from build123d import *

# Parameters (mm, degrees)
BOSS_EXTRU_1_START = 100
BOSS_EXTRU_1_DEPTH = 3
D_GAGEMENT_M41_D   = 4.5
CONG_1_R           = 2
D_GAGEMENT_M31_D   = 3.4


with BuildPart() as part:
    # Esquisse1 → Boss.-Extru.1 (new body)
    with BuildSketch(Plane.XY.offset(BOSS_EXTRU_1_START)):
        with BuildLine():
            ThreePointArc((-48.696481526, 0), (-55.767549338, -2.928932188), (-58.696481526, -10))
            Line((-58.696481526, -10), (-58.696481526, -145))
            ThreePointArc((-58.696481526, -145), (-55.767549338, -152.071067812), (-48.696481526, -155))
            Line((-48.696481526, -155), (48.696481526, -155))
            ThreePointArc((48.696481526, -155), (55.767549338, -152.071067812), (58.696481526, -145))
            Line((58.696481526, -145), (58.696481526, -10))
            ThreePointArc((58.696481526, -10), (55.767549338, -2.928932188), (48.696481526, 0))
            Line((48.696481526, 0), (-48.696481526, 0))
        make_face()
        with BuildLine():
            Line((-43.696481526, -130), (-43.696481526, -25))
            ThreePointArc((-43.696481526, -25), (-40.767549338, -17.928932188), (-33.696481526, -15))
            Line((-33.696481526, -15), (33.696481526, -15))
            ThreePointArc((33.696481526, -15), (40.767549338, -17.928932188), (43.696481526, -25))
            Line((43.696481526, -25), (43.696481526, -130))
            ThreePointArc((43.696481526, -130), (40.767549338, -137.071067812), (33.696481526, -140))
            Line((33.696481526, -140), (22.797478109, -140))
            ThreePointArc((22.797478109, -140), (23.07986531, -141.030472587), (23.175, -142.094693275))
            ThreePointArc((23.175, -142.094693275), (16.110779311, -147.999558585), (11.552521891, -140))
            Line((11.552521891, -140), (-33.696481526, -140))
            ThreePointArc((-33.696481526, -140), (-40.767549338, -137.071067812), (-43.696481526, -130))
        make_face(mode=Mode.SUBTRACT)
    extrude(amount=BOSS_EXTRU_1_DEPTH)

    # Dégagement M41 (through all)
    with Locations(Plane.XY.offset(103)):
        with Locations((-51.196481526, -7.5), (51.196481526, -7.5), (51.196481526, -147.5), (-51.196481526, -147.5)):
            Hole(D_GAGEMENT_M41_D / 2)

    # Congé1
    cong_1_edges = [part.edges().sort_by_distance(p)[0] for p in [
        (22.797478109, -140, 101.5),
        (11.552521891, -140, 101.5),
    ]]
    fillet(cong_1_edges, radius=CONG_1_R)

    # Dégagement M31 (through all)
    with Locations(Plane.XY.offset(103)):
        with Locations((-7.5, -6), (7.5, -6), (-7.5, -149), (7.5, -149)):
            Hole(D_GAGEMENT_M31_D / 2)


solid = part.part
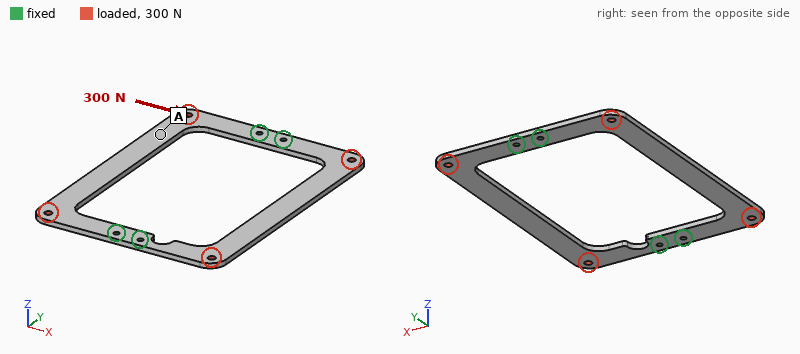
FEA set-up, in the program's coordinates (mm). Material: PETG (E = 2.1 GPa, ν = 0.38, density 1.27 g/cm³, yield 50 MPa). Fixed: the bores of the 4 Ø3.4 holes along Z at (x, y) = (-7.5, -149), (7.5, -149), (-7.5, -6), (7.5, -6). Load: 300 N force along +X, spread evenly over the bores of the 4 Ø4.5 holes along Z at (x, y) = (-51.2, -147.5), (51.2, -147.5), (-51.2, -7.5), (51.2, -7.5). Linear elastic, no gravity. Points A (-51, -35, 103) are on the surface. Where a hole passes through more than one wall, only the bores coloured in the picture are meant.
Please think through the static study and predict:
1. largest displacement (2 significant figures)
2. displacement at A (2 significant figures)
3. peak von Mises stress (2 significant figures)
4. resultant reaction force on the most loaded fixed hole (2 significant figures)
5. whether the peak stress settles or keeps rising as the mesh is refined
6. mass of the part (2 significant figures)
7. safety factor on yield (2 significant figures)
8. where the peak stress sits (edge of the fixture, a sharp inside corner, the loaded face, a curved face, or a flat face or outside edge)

72 µm
21 µm
9.2 MPa
78 N
settles
27 g
5.5
a curved face
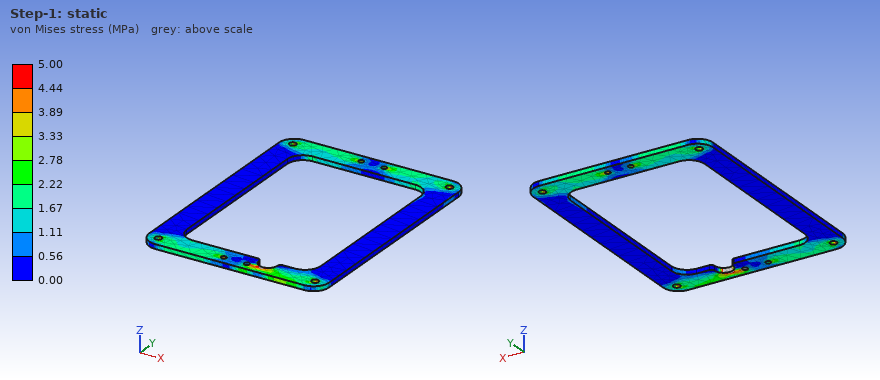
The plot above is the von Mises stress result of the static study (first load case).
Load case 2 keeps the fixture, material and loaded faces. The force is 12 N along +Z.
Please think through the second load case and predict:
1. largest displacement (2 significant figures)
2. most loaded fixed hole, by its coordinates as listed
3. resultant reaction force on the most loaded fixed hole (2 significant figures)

2.1 mm
(-7.5, -149)
3.8 N
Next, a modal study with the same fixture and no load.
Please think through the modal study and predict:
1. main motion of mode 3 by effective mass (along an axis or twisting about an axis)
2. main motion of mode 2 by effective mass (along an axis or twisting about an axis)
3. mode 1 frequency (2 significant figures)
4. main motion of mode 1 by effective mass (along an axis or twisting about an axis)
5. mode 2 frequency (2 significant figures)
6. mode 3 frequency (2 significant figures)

twisting about X
along Z
86 Hz
along Z
96 Hz
200 Hz
